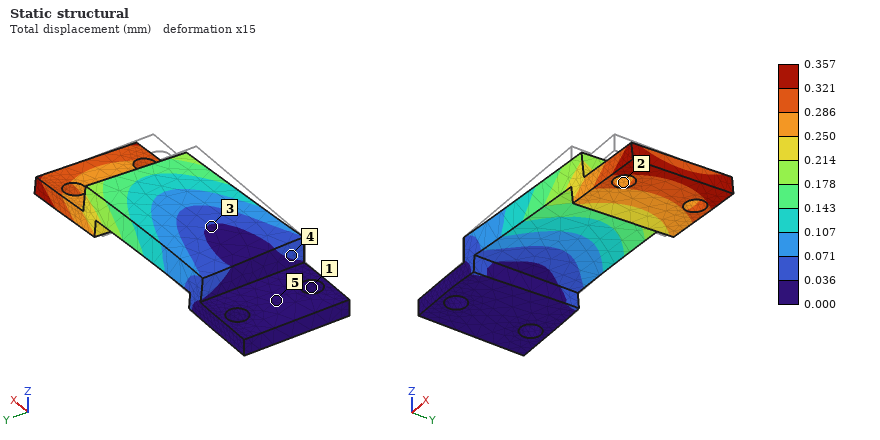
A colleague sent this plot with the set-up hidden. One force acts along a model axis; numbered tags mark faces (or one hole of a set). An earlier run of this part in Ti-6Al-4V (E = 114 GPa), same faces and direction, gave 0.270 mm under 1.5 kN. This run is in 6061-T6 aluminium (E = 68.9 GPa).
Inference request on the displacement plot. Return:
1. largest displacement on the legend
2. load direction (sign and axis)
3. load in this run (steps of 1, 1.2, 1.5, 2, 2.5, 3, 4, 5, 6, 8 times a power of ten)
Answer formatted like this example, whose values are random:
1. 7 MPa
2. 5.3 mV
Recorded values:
1. 0.357 mm
2. +Y
3. 1.2 kN
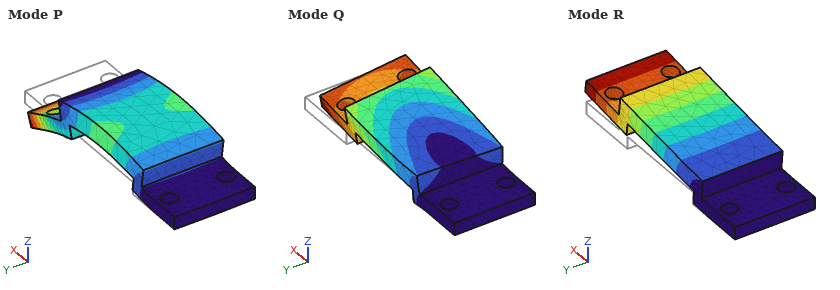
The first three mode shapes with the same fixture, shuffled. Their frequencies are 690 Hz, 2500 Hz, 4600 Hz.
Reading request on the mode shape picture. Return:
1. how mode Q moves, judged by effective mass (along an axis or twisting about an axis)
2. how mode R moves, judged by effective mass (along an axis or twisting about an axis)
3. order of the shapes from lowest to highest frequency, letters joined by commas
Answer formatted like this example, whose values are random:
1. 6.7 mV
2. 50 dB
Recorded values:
1. along Y
2. along Z
3. R, Q, P
